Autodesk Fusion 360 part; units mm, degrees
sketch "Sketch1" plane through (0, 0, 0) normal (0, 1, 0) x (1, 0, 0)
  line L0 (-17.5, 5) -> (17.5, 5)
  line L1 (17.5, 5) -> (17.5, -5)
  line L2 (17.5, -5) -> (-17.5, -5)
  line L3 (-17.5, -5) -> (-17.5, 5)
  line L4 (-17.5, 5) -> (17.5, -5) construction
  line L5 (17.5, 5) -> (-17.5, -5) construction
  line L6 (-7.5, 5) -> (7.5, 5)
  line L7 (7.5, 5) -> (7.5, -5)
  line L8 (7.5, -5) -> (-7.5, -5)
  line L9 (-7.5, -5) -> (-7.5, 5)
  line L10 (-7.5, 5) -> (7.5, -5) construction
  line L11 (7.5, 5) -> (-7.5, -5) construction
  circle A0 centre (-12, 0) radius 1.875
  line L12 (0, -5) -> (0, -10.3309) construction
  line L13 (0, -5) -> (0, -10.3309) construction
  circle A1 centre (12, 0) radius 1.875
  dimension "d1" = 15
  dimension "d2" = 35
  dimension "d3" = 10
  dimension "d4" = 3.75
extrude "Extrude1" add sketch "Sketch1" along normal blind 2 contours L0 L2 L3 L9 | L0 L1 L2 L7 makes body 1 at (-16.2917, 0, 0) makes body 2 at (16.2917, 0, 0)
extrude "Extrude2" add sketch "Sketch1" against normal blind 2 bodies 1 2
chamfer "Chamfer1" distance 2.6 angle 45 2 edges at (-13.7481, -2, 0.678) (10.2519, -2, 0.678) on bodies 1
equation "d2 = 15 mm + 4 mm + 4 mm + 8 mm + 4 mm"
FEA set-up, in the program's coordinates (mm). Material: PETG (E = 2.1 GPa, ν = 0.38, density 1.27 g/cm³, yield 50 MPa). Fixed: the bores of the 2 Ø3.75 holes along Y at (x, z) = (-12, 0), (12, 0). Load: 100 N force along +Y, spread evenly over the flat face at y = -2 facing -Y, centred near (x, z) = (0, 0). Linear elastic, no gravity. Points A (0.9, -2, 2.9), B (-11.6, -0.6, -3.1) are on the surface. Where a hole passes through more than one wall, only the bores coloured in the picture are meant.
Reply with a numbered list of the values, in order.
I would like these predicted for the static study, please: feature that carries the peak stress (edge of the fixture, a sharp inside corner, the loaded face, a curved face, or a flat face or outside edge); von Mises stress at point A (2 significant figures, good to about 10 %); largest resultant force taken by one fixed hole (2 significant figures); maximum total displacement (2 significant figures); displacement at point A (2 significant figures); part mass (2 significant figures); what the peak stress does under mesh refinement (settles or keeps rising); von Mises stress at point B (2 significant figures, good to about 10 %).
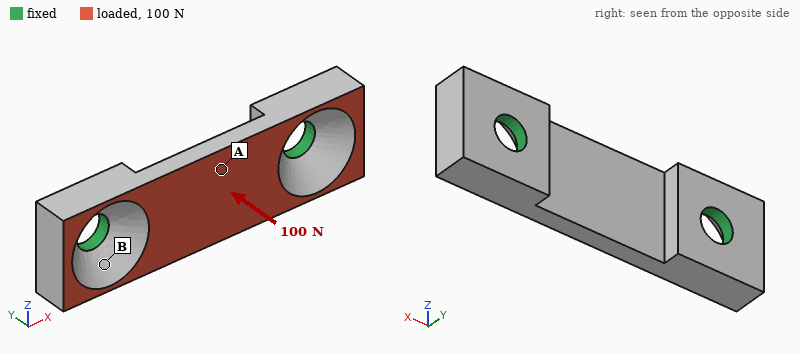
1. edge of the fixture
2. 11 MPa
3. 69 N
4. 0.13 mm
5. 0.11 mm
6. 1.1 g
7. keeps rising
8. 3.2 MPa
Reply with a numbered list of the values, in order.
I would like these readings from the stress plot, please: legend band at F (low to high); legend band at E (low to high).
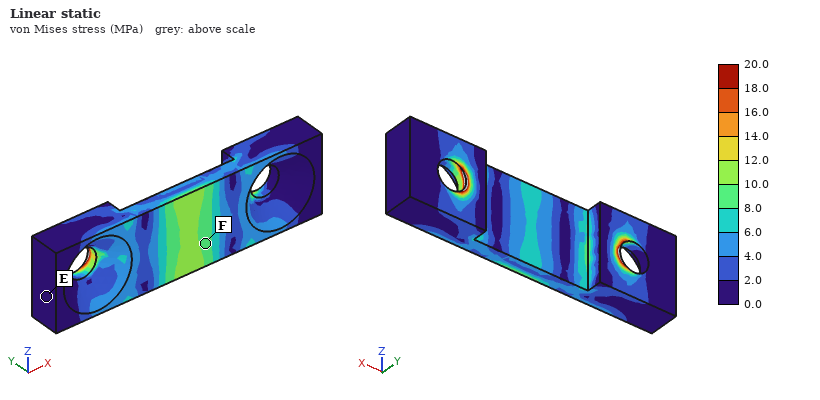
1. 8.0 to 10.0 MPa
2. 0.0 to 2.0 MPa
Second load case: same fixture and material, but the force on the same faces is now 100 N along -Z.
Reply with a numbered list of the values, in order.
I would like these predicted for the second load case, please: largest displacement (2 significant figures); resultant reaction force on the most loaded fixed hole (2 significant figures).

1. 0.11 mm
2. 50 N
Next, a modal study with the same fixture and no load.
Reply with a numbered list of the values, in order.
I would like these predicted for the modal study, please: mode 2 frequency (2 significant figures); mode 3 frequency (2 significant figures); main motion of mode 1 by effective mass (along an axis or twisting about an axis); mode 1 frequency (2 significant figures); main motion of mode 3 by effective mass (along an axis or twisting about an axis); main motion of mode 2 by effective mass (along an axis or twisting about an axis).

1. 7400 Hz
2. 10 kHz
3. along Y
4. 6800 Hz
5. along X
6. along Z
